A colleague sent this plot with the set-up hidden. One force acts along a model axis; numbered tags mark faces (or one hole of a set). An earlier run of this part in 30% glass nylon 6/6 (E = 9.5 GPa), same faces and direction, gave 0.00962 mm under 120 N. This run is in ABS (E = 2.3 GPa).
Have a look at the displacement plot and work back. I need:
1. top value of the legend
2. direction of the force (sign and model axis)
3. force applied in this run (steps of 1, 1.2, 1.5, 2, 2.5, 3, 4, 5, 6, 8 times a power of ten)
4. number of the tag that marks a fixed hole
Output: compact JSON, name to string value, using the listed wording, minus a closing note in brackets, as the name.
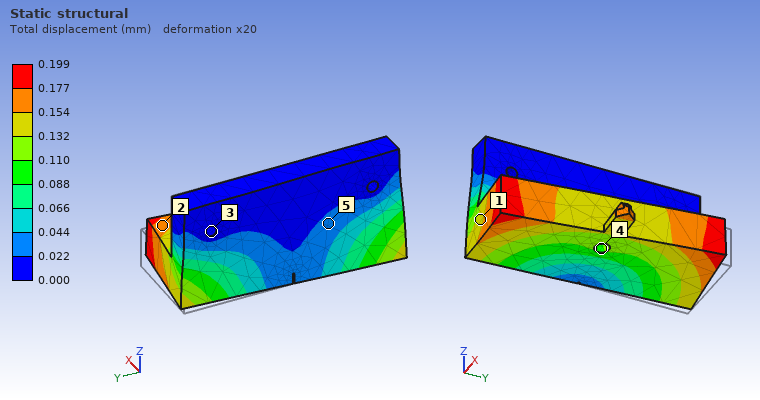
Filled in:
{"top value of the legend": "0.199 mm", "direction of the force": "-Y", "force applied in this run": "600 N", "number of the tag that marks a fixed hole": "3"}
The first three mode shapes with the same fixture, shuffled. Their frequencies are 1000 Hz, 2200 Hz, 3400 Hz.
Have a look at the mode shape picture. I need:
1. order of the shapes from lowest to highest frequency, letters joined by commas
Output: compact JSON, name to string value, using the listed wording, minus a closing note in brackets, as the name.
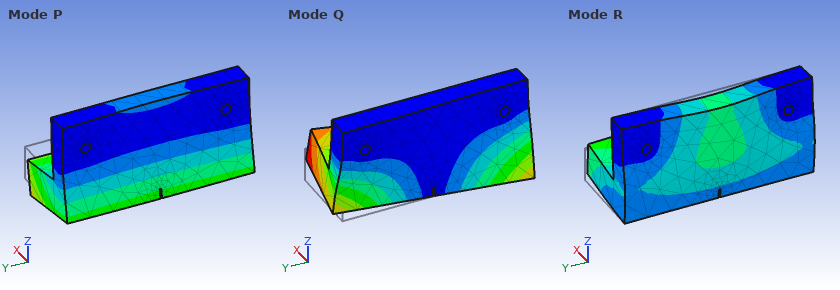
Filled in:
{"order of the shapes from lowest to highest frequency, letters joined by commas": "P, Q, R"}
